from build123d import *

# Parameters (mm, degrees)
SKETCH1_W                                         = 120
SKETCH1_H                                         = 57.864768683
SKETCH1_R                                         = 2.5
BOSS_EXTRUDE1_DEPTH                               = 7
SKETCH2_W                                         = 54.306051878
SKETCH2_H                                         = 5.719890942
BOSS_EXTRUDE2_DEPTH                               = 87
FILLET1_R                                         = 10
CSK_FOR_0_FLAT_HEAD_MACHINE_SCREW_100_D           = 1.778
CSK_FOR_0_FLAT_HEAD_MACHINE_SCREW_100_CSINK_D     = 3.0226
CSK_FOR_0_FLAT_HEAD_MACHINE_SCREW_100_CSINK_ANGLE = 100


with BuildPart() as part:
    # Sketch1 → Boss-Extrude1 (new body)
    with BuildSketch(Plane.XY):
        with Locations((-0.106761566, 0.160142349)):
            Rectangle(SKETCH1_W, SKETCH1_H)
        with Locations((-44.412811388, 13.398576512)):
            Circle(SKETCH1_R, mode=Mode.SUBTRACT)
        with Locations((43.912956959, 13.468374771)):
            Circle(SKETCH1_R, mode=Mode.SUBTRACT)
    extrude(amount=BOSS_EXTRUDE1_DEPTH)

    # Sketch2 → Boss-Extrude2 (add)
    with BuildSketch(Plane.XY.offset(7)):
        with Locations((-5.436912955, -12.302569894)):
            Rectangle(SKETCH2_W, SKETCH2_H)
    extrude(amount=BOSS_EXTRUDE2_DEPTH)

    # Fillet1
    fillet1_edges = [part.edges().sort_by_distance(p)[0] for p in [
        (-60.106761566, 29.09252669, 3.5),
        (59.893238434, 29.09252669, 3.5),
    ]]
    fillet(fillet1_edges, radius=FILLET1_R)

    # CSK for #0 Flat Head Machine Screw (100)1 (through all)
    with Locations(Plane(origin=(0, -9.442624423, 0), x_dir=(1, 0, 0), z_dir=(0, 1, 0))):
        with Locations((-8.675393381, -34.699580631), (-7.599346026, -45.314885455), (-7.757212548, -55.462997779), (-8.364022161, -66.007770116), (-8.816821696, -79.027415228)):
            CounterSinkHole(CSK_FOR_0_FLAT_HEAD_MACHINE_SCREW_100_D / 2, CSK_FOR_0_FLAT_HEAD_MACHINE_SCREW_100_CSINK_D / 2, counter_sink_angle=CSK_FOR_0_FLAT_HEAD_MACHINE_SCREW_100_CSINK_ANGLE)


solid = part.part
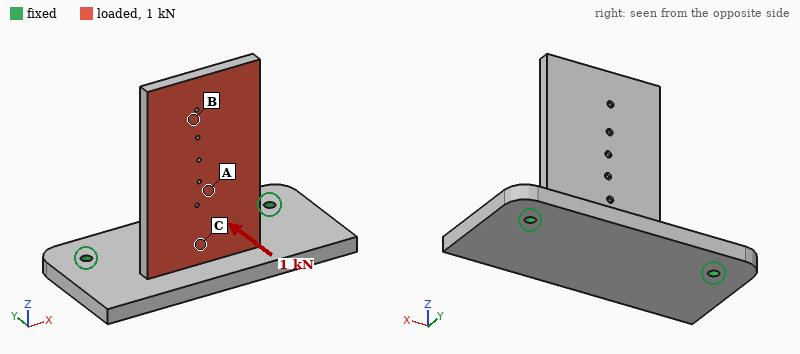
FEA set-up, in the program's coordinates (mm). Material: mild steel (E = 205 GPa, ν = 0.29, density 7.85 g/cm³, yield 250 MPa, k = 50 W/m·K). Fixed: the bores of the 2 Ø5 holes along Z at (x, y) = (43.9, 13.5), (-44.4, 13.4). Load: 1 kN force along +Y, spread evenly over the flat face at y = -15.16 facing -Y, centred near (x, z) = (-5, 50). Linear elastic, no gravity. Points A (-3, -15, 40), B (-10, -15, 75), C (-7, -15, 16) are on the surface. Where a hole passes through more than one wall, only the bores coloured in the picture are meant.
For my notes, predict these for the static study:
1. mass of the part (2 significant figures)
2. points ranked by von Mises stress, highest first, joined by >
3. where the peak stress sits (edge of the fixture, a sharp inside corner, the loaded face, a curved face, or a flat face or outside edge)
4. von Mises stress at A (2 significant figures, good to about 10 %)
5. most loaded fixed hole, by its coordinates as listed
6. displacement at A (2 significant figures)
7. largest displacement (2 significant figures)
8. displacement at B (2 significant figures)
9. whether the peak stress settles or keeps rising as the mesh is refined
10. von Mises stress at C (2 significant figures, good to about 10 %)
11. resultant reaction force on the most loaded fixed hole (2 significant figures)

590 g
C > A > B
edge of the fixture
53 MPa
(-44.4, 13.4)
0.22 mm
0.74 mm
0.55 mm
keeps rising
100 MPa
610 N
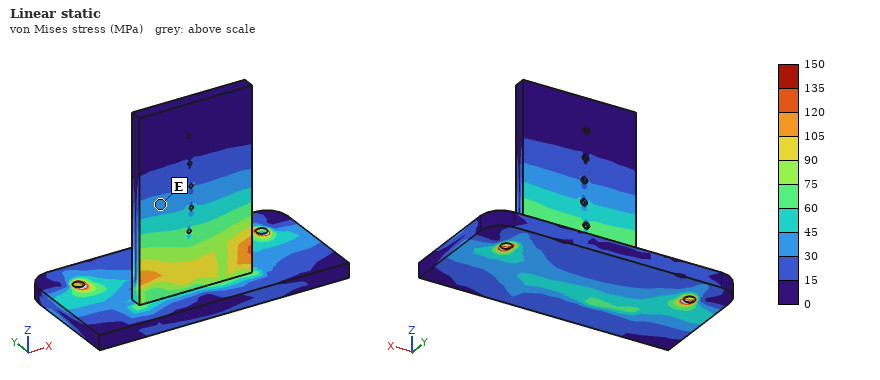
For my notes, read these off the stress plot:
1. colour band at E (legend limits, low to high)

30 to 45 MPa
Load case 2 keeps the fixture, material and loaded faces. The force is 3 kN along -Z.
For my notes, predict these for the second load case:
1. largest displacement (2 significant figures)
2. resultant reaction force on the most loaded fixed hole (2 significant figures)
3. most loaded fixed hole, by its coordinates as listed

0.42 mm
1.7 kN
(-44.4, 13.4)
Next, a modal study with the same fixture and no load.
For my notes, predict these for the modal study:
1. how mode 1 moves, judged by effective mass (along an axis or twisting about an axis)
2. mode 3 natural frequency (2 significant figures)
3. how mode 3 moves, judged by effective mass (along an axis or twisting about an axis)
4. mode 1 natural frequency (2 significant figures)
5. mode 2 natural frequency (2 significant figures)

along Y
1800 Hz
along Z
500 Hz
1600 Hz
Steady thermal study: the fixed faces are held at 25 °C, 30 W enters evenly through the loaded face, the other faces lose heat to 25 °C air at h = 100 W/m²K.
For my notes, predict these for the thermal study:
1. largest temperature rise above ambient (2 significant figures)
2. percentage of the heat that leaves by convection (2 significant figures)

36 K
83 %
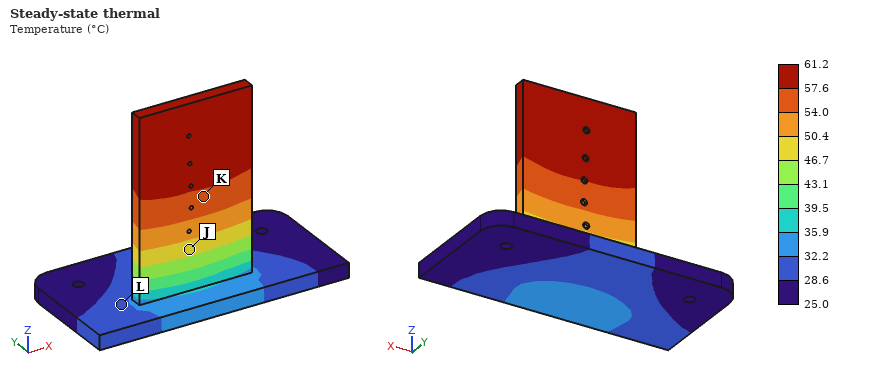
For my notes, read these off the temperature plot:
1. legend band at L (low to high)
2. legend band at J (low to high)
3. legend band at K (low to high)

28.6 to 32.2 °C
46.7 to 50.4 °C
54.0 to 57.6 °C
